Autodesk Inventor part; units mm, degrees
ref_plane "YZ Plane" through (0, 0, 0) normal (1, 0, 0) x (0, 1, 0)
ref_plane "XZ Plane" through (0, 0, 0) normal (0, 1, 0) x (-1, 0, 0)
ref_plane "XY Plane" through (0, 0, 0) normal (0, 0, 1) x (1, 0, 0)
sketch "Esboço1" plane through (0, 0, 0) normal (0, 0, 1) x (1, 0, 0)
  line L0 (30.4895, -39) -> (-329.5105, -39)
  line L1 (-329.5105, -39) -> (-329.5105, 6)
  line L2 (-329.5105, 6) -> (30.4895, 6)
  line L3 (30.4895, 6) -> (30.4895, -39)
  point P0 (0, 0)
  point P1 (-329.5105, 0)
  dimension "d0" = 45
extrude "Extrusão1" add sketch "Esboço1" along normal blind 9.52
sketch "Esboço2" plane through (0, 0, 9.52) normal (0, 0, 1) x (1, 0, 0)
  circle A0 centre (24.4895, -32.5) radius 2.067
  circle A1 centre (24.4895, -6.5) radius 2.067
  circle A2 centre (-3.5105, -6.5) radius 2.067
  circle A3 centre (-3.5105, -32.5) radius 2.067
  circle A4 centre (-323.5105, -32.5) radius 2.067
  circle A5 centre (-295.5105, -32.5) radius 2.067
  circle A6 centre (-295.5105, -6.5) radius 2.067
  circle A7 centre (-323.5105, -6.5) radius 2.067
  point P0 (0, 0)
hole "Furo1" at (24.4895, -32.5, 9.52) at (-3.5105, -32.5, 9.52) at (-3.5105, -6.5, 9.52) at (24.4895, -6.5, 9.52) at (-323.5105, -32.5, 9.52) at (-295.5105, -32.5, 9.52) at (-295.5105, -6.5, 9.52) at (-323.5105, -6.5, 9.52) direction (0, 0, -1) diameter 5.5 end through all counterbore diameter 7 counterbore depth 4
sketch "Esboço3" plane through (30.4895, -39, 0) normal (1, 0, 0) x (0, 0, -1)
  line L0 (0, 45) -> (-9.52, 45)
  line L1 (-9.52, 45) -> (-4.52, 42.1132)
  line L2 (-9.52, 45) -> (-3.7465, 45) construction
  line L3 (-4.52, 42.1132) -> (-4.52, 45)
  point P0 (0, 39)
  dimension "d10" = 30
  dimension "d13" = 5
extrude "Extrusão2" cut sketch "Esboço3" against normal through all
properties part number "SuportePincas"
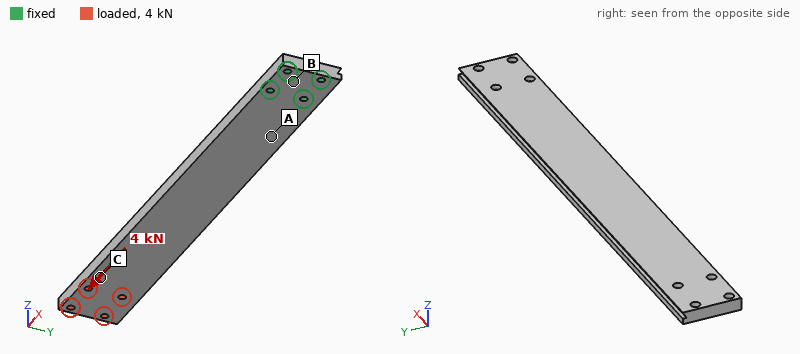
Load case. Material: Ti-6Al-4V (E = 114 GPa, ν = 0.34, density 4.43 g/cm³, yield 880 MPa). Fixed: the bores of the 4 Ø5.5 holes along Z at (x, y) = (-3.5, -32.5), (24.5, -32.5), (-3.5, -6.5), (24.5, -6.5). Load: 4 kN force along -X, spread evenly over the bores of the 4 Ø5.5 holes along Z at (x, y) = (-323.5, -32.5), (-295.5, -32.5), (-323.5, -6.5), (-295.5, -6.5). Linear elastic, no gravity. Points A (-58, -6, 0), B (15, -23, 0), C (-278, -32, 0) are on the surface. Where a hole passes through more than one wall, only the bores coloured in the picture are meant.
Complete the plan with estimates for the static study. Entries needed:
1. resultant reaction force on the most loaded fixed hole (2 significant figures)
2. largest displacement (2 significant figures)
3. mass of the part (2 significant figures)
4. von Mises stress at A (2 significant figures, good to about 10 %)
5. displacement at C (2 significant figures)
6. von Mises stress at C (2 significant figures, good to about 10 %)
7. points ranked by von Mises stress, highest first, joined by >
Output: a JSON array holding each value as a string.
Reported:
["1.8 kN", "1.1 mm", "660 g", "19 MPa", "0.81 mm", "24 MPa", "C > A > B"]
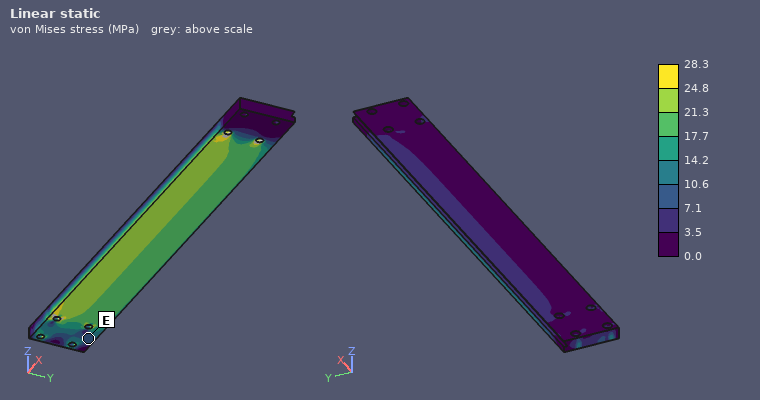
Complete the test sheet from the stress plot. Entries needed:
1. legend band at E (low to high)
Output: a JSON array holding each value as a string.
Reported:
["7.1 to 10.6 MPa"]
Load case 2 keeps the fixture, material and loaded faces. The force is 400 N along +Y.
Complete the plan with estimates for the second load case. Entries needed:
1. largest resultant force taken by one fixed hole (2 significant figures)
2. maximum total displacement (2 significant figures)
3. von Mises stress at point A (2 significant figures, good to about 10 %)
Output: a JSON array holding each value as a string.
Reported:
["3.5 kN", "0.58 mm", "16 MPa"]
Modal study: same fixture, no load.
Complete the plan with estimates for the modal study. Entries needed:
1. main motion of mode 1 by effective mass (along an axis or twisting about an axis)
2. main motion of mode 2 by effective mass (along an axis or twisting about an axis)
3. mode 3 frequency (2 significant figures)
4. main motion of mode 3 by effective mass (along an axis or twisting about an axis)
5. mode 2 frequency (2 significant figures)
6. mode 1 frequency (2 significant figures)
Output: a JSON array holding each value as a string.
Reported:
["along Z", "along Y", "450 Hz", "along Z", "330 Hz", "73 Hz"]
